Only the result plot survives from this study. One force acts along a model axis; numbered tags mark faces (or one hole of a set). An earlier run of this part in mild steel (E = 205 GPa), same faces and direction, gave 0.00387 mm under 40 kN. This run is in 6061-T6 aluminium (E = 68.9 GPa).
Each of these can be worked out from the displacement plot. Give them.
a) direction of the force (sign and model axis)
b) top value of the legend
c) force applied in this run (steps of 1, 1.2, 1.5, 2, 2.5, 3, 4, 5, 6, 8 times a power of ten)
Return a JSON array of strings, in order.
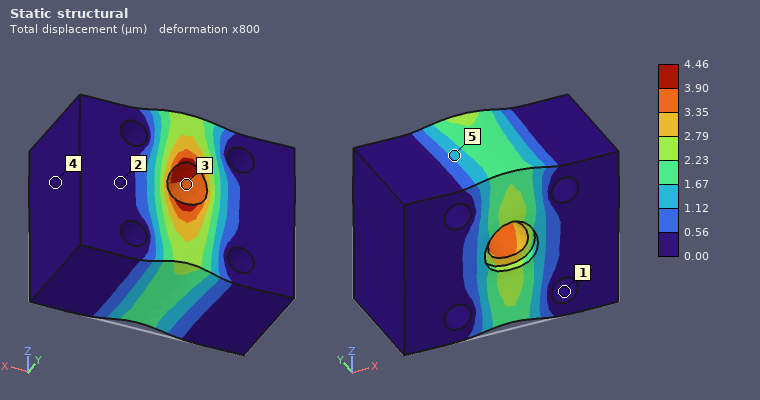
["+Z", "4.46 µm", "15 kN"]
